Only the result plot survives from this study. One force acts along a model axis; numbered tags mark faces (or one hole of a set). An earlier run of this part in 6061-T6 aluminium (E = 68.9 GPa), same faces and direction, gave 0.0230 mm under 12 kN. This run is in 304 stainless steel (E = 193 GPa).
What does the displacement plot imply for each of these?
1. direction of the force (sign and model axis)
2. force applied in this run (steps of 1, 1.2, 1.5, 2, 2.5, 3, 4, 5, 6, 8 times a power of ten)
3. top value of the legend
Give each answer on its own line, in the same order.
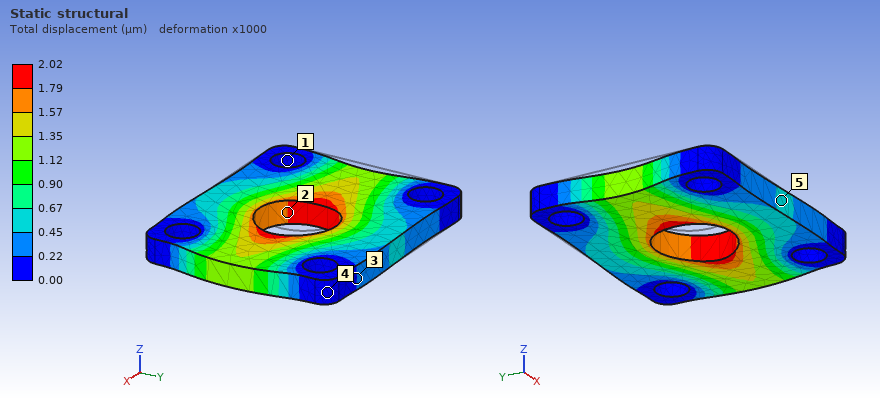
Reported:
+X
3 kN
2.02 µm
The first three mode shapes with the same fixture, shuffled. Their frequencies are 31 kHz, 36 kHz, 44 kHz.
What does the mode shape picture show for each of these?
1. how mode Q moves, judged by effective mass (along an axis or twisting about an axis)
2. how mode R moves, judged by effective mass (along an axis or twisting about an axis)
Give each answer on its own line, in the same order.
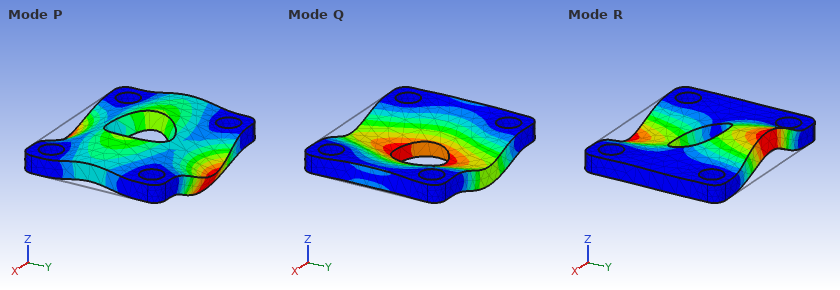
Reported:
along Z
twisting about X
